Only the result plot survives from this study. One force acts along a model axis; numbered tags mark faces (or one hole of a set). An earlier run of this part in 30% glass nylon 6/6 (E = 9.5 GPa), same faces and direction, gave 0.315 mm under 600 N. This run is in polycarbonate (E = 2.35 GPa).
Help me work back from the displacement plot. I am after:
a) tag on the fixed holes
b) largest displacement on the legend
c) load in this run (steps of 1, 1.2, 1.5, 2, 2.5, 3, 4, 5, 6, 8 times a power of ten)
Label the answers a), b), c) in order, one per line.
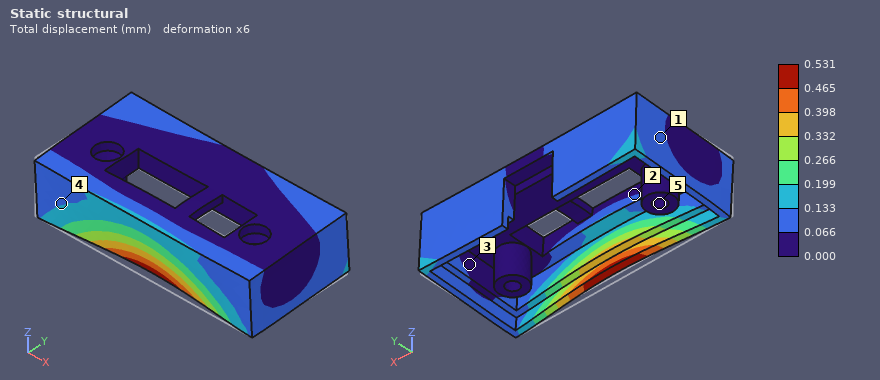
a) 5
b) 0.531 mm
c) 250 N
